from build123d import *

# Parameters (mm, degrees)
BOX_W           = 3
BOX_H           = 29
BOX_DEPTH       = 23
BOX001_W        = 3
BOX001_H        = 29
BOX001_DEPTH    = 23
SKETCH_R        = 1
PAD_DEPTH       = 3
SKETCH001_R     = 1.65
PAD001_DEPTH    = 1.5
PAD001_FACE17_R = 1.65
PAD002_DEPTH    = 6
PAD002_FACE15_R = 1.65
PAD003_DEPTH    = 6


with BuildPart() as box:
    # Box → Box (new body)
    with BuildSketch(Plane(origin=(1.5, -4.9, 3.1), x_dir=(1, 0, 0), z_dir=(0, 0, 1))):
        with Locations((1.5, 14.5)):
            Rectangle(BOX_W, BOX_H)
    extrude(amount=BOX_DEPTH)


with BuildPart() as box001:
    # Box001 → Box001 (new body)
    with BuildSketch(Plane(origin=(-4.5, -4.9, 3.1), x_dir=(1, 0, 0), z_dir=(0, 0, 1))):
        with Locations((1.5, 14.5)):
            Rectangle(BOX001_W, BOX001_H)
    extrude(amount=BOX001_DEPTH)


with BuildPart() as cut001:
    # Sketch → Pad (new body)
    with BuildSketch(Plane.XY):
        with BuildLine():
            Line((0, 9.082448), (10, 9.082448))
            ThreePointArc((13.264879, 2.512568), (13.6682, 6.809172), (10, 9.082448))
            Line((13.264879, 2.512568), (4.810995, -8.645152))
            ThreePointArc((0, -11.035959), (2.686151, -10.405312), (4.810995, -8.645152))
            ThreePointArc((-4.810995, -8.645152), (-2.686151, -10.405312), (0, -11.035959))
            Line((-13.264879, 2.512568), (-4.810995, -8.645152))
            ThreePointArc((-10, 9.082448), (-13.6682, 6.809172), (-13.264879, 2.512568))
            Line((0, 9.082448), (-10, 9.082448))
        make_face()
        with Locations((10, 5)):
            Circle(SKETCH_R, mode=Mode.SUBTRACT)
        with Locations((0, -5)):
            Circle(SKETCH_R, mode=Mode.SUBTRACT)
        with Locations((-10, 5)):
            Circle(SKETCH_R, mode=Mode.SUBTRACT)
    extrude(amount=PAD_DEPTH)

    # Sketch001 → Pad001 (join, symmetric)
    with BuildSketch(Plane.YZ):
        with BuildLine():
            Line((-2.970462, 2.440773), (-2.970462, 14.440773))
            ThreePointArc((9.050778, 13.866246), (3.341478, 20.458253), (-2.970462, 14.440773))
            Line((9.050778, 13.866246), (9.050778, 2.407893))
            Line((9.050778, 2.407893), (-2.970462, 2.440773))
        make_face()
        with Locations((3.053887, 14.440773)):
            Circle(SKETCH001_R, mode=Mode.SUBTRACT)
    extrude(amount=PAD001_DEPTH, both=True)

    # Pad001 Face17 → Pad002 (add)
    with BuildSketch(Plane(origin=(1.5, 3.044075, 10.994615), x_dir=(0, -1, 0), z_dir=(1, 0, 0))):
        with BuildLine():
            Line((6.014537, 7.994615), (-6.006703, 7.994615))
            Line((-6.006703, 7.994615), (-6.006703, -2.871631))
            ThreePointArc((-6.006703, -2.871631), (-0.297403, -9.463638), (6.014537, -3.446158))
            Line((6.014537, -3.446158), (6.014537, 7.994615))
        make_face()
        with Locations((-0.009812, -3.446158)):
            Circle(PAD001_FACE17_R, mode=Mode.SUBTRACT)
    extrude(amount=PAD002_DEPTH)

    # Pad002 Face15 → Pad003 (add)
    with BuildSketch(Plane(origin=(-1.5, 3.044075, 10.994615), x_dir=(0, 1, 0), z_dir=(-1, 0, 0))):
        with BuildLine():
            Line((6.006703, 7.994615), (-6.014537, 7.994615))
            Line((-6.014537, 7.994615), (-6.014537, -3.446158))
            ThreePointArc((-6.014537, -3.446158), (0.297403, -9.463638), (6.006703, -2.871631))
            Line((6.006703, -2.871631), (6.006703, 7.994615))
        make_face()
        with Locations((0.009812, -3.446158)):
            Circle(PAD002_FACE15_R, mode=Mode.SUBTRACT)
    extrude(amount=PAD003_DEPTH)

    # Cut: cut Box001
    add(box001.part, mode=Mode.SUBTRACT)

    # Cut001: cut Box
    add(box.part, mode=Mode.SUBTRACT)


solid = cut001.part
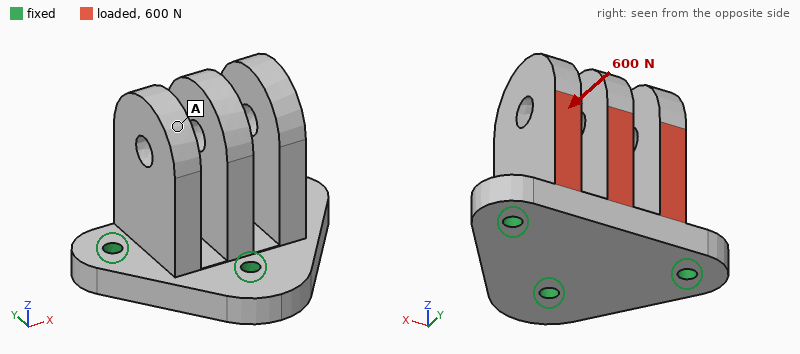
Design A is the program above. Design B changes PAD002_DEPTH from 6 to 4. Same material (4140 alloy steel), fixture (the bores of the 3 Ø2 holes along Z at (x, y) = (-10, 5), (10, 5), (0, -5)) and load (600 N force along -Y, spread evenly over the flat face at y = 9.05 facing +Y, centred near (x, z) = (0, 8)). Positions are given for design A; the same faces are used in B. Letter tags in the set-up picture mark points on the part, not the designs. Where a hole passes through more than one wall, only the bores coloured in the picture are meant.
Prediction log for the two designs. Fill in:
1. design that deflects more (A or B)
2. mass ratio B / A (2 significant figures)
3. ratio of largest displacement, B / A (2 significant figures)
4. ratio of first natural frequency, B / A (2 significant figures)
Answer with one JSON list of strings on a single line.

["B", "0.87", "1.2", "0.44"]
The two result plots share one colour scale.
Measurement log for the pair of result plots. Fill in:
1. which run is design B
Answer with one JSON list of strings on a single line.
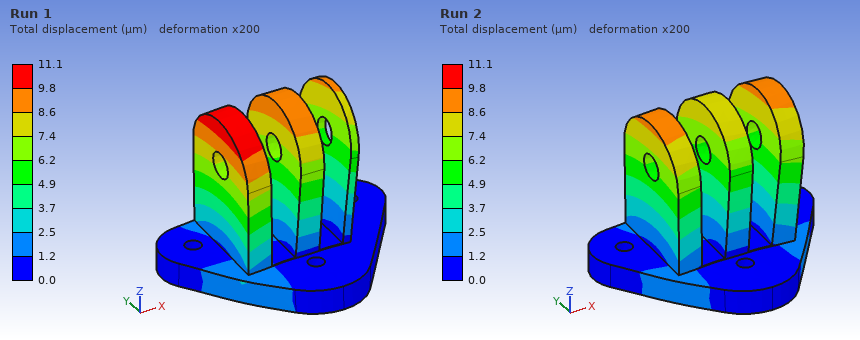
["Run 1"]
